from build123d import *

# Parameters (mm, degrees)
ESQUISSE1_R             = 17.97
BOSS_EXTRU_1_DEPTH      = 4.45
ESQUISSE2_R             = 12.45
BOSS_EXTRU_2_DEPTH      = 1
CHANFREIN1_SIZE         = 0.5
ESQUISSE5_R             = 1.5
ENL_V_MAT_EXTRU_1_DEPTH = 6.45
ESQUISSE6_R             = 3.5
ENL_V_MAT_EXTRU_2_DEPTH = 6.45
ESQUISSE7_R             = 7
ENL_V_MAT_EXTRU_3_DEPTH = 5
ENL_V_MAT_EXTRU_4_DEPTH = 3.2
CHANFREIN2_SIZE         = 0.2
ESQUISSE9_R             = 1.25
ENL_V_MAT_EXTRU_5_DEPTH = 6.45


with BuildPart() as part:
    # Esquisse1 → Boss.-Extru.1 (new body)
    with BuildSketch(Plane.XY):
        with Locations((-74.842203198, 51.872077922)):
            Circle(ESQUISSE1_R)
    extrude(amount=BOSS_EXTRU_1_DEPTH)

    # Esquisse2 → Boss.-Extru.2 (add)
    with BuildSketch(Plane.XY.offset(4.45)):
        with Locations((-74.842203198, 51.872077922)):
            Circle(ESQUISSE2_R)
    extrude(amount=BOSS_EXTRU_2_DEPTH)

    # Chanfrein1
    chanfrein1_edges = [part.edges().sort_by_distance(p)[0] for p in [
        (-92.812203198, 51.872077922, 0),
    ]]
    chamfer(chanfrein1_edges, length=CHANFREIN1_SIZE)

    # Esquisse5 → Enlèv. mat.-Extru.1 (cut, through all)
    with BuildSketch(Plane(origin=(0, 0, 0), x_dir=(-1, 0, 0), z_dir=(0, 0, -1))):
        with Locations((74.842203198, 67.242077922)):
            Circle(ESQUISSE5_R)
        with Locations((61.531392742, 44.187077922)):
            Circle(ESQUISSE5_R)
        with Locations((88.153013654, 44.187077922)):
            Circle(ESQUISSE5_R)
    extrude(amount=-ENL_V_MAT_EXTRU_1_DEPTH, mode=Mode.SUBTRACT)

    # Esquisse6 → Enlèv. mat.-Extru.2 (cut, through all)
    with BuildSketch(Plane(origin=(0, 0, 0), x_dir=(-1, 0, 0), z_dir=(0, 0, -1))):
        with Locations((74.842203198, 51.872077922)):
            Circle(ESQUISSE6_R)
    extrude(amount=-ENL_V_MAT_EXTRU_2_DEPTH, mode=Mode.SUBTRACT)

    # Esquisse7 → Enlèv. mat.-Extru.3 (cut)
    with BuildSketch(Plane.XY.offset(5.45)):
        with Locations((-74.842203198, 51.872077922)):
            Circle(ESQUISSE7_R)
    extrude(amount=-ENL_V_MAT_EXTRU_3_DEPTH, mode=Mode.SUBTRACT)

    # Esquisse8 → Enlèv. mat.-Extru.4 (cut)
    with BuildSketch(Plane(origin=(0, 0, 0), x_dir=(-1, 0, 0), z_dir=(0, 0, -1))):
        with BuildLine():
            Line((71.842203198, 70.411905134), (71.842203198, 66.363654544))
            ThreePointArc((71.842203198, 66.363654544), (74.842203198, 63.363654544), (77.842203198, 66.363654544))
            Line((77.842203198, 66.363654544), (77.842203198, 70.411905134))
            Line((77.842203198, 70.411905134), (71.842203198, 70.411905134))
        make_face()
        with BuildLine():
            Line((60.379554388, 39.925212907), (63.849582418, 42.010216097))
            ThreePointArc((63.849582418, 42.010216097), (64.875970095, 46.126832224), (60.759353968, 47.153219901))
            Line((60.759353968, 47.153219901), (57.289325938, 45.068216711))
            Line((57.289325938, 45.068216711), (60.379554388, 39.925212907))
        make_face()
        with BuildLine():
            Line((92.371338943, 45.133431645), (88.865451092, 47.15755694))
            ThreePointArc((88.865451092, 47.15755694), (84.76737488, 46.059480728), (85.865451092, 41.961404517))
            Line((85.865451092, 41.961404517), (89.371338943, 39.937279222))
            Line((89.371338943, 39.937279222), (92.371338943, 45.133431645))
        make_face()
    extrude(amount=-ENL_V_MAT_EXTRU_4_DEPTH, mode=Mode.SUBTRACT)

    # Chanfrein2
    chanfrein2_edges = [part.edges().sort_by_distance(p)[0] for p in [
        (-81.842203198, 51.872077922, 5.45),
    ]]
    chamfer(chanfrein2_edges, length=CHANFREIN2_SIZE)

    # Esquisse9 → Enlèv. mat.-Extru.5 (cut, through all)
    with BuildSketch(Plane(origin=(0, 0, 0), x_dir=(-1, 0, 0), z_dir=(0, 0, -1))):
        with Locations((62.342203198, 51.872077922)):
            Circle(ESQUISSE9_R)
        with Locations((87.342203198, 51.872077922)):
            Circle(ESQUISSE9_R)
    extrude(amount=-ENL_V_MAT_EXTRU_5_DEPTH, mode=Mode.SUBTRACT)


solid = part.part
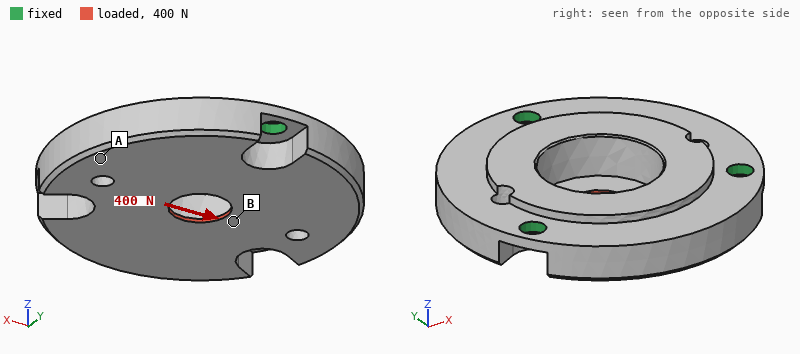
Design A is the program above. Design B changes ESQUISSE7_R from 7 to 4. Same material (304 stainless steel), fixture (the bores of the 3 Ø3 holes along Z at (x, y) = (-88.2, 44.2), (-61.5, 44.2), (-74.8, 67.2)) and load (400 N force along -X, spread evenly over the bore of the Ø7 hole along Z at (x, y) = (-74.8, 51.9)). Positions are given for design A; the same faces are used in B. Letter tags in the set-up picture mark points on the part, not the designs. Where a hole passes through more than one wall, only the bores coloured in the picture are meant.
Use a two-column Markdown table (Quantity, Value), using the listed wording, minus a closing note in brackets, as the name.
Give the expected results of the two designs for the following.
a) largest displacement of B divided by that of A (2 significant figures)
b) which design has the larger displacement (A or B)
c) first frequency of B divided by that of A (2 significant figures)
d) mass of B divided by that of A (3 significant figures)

| Quantity | Value |
|---|---|
| largest displacement of B divided by that of A | 0.80 |
| which design has the larger displacement | A |
| first frequency of B divided by that of A | 1.0 |
| mass of B divided by that of A | 1.14 |
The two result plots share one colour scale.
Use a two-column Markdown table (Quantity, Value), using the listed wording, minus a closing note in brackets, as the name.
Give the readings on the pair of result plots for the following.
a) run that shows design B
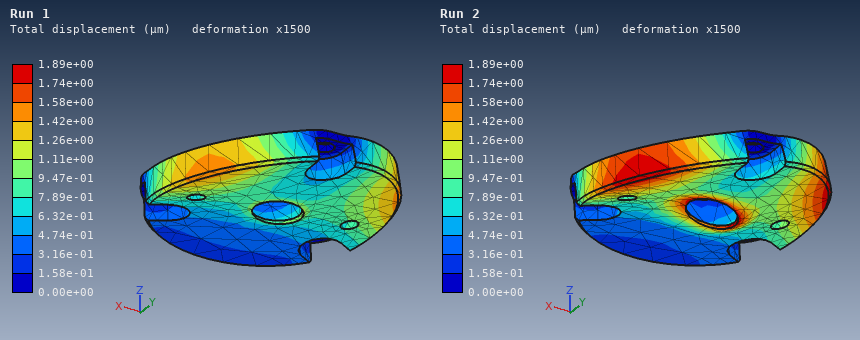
| Quantity | Value |
|---|---|
| run that shows design B | Run 1 |
